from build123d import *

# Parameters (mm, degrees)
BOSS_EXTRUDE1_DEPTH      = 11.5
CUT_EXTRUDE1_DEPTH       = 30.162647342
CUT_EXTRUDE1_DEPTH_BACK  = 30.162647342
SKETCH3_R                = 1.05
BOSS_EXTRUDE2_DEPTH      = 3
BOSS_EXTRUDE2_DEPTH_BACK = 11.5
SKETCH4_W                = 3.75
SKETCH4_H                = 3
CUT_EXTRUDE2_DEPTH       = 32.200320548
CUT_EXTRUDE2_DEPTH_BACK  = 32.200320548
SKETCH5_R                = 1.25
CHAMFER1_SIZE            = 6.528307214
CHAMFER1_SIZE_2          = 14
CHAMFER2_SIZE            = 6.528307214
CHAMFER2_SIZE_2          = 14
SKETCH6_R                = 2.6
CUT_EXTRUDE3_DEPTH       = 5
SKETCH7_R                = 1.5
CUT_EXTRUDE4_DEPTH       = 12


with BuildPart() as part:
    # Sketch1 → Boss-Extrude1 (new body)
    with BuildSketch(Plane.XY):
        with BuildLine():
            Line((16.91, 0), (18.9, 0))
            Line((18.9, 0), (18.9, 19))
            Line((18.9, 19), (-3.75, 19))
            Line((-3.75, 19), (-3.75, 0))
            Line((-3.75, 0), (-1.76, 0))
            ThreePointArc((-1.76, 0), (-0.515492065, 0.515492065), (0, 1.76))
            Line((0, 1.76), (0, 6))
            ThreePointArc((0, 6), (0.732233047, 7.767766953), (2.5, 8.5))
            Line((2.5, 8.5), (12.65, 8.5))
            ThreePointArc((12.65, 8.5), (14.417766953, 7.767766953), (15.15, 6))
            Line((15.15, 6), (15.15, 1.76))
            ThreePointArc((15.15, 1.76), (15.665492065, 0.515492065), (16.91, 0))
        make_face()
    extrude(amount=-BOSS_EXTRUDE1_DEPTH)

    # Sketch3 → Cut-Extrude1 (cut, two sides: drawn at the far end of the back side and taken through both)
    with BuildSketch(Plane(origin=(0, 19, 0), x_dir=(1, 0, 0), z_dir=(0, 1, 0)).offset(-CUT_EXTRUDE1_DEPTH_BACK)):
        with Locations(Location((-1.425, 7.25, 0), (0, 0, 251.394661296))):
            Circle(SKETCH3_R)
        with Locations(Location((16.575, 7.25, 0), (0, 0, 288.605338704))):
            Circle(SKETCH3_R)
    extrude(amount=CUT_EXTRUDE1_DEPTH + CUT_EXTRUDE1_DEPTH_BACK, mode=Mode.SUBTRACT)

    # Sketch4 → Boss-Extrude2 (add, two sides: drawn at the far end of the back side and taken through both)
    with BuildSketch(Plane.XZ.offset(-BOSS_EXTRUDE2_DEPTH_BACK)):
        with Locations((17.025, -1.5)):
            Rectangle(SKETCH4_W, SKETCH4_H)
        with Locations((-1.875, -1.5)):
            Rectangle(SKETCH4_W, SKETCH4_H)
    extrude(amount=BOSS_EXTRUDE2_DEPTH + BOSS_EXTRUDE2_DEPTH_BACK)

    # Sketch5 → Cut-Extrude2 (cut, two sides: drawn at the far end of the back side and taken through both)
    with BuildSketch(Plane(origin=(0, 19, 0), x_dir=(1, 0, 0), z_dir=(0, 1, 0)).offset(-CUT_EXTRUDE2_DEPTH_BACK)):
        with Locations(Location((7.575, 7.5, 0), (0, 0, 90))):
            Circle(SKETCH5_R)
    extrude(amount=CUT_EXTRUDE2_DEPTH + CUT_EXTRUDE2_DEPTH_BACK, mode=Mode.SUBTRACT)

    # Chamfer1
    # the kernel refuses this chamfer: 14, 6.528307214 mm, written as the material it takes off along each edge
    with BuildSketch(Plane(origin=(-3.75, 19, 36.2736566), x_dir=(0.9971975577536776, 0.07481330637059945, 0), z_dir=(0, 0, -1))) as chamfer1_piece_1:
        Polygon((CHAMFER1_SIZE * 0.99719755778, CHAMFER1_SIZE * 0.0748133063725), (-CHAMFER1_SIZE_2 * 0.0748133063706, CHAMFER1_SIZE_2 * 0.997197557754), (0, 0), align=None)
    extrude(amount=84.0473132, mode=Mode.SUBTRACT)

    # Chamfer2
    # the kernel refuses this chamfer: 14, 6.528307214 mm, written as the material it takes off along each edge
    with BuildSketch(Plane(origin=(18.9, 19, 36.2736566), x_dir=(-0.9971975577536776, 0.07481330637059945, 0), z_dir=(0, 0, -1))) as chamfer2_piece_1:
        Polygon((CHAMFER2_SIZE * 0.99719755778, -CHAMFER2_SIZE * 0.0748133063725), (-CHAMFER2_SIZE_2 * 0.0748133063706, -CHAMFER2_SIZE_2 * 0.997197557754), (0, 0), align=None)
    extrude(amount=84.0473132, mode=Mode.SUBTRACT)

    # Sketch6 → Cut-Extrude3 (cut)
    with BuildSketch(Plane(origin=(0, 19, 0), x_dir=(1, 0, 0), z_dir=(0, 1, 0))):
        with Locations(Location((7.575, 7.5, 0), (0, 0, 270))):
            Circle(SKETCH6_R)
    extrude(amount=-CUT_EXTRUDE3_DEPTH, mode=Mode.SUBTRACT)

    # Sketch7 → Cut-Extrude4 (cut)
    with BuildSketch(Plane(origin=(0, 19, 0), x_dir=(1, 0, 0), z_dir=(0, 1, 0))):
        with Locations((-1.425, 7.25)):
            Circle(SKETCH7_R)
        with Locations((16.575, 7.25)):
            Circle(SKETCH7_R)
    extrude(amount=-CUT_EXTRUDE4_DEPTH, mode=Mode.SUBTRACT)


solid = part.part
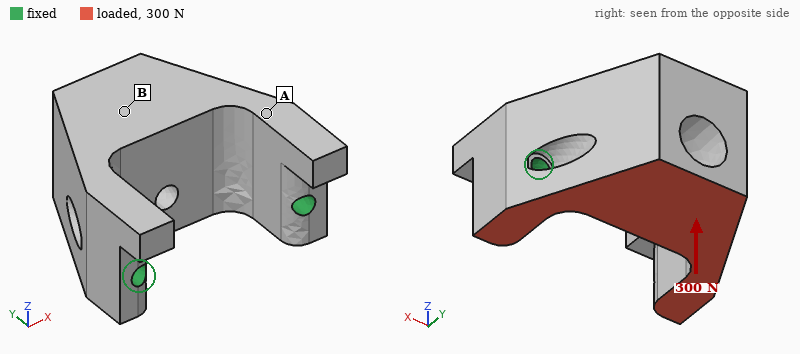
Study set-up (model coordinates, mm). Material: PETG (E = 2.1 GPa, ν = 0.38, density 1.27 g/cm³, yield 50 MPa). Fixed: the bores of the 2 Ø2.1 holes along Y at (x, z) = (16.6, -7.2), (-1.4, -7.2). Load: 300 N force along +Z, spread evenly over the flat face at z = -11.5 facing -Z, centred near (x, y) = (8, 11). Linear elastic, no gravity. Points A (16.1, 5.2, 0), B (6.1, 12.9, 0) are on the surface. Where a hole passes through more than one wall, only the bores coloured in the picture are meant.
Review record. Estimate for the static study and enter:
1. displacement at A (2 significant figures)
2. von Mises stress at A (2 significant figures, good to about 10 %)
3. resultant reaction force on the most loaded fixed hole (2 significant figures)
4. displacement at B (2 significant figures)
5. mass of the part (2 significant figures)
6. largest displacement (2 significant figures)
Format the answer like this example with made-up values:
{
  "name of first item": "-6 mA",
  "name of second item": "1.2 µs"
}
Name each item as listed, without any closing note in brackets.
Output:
{
  "displacement at A": "0.075 mm",
  "von Mises stress at A": "11 MPa",
  "resultant reaction force on the most loaded fixed hole": "150 N",
  "displacement at B": "0.18 mm",
  "mass of the part": "2.9 g",
  "largest displacement": "0.27 mm"
}
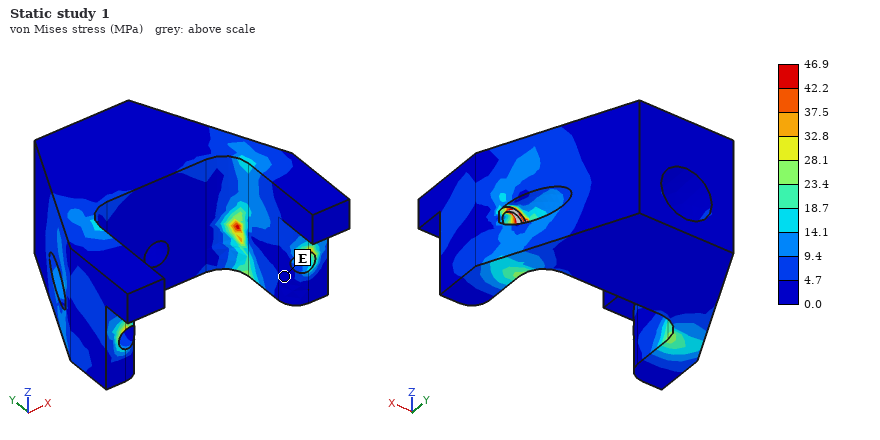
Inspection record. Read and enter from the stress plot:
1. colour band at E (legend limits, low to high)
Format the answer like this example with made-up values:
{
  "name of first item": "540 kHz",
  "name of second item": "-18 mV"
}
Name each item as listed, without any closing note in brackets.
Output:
{
  "colour band at E": "0.0 to 4.7 MPa"
}
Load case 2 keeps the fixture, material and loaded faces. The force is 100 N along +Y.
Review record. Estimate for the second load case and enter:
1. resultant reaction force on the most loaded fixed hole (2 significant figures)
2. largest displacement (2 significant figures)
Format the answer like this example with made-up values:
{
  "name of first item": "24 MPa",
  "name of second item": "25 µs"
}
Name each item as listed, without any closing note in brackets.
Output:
{
  "resultant reaction force on the most loaded fixed hole": "53 N",
  "largest displacement": "69 µm"
}
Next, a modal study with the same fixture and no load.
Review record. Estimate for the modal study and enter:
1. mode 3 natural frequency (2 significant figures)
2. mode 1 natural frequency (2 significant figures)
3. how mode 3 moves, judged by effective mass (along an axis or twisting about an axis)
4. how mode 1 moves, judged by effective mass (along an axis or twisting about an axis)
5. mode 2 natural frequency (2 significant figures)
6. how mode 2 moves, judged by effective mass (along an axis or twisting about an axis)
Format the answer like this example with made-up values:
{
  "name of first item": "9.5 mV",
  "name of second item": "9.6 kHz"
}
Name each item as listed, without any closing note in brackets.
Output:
{
  "mode 3 natural frequency": "9800 Hz",
  "mode 1 natural frequency": "3800 Hz",
  "how mode 3 moves, judged by effective mass": "along Y",
  "how mode 1 moves, judged by effective mass": "along Z",
  "mode 2 natural frequency": "6700 Hz",
  "how mode 2 moves, judged by effective mass": "along X"
}
